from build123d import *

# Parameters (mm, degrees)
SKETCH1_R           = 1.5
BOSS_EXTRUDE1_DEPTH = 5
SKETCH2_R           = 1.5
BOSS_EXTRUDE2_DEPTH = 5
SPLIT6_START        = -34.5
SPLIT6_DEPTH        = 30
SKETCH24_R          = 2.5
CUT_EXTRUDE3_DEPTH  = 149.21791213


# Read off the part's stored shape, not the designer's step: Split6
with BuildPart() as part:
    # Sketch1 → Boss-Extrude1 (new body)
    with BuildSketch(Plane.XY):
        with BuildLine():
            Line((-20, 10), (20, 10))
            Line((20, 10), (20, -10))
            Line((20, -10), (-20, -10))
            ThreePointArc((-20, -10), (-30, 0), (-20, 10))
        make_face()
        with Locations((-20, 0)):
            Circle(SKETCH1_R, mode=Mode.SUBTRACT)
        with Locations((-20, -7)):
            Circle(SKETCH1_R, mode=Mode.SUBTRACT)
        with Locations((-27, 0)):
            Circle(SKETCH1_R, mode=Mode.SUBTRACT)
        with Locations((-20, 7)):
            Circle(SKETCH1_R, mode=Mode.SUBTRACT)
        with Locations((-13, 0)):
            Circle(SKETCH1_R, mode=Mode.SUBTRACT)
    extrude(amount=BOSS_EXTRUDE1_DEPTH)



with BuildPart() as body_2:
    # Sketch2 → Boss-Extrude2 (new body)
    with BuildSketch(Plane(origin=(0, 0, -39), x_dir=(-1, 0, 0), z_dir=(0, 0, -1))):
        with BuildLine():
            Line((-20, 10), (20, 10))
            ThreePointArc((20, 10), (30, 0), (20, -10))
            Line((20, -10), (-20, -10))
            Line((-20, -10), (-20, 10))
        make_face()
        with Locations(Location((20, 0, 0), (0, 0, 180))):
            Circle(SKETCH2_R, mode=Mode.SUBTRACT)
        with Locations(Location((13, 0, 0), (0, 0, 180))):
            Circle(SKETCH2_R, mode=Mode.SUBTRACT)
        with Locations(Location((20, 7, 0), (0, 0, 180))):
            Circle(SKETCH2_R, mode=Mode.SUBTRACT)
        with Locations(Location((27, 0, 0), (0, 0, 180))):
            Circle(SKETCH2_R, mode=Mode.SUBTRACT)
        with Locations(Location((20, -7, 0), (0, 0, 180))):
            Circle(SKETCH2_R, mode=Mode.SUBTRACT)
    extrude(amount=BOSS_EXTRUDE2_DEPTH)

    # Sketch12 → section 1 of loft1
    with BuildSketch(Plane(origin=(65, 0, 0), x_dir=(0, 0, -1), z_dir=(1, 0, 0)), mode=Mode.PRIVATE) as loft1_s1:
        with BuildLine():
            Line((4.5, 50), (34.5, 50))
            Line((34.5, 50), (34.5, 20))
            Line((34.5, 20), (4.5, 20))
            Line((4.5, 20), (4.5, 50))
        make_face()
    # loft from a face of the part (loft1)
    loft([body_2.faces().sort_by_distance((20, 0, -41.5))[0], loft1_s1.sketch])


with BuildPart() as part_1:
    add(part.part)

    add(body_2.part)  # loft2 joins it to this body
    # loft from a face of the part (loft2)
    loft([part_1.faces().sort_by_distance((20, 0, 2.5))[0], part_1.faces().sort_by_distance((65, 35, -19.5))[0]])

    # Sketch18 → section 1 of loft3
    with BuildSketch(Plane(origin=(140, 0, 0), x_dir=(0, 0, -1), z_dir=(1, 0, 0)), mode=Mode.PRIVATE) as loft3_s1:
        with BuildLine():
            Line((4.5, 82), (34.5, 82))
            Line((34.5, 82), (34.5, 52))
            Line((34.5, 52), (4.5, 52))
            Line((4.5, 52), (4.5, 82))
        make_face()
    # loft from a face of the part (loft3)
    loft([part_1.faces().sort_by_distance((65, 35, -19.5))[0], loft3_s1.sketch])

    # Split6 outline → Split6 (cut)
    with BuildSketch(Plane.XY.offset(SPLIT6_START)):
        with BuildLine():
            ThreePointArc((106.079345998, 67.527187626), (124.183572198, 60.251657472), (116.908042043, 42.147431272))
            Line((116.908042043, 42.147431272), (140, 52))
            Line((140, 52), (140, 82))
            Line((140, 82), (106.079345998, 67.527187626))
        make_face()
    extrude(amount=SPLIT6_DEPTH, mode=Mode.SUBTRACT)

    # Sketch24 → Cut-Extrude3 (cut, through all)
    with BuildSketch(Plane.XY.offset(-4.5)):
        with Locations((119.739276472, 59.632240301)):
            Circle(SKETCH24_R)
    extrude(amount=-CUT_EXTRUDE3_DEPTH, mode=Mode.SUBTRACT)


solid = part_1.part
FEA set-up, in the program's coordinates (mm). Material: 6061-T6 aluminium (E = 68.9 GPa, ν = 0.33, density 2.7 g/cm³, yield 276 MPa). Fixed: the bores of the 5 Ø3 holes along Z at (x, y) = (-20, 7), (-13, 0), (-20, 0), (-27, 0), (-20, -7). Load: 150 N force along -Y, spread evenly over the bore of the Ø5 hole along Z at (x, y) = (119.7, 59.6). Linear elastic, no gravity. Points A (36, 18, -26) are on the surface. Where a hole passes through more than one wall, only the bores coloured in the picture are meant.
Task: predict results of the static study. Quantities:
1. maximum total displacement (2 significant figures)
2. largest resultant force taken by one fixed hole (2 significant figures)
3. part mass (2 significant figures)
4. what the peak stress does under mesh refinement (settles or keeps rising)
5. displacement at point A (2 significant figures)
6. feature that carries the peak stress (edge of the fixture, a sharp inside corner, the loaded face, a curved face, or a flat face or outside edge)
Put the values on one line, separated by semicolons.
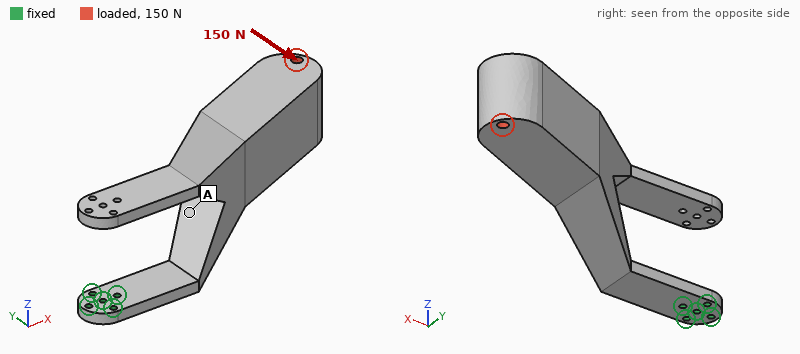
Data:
0.83 mm; 1.0 kN; 250 g; keeps rising; 0.23 mm; edge of the fixture
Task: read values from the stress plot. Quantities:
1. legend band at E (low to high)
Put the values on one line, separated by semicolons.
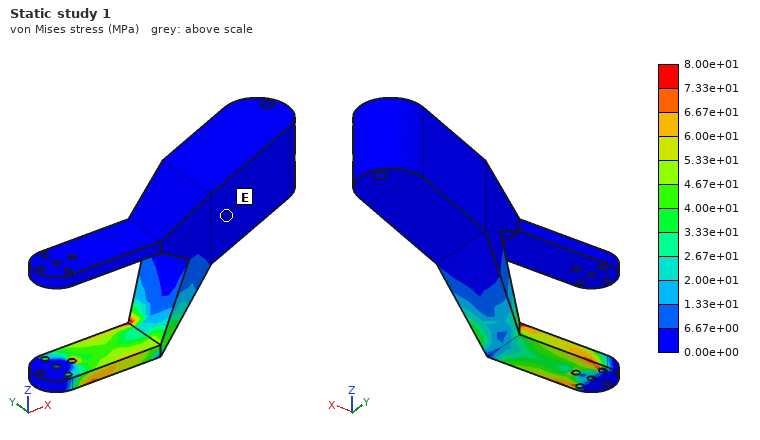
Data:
0.00e+00 to 6.67e+00 MPa
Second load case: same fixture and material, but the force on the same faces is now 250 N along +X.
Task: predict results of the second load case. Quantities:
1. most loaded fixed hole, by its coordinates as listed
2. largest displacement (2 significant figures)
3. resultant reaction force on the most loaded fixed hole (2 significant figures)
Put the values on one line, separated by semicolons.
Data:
(-20, 7); 2.1 mm; 840 N
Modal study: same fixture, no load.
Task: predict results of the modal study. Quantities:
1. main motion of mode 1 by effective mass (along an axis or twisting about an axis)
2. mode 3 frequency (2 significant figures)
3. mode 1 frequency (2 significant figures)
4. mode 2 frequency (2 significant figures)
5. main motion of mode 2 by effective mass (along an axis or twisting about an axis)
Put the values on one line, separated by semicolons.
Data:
along Z; 430 Hz; 74 Hz; 200 Hz; along Y
